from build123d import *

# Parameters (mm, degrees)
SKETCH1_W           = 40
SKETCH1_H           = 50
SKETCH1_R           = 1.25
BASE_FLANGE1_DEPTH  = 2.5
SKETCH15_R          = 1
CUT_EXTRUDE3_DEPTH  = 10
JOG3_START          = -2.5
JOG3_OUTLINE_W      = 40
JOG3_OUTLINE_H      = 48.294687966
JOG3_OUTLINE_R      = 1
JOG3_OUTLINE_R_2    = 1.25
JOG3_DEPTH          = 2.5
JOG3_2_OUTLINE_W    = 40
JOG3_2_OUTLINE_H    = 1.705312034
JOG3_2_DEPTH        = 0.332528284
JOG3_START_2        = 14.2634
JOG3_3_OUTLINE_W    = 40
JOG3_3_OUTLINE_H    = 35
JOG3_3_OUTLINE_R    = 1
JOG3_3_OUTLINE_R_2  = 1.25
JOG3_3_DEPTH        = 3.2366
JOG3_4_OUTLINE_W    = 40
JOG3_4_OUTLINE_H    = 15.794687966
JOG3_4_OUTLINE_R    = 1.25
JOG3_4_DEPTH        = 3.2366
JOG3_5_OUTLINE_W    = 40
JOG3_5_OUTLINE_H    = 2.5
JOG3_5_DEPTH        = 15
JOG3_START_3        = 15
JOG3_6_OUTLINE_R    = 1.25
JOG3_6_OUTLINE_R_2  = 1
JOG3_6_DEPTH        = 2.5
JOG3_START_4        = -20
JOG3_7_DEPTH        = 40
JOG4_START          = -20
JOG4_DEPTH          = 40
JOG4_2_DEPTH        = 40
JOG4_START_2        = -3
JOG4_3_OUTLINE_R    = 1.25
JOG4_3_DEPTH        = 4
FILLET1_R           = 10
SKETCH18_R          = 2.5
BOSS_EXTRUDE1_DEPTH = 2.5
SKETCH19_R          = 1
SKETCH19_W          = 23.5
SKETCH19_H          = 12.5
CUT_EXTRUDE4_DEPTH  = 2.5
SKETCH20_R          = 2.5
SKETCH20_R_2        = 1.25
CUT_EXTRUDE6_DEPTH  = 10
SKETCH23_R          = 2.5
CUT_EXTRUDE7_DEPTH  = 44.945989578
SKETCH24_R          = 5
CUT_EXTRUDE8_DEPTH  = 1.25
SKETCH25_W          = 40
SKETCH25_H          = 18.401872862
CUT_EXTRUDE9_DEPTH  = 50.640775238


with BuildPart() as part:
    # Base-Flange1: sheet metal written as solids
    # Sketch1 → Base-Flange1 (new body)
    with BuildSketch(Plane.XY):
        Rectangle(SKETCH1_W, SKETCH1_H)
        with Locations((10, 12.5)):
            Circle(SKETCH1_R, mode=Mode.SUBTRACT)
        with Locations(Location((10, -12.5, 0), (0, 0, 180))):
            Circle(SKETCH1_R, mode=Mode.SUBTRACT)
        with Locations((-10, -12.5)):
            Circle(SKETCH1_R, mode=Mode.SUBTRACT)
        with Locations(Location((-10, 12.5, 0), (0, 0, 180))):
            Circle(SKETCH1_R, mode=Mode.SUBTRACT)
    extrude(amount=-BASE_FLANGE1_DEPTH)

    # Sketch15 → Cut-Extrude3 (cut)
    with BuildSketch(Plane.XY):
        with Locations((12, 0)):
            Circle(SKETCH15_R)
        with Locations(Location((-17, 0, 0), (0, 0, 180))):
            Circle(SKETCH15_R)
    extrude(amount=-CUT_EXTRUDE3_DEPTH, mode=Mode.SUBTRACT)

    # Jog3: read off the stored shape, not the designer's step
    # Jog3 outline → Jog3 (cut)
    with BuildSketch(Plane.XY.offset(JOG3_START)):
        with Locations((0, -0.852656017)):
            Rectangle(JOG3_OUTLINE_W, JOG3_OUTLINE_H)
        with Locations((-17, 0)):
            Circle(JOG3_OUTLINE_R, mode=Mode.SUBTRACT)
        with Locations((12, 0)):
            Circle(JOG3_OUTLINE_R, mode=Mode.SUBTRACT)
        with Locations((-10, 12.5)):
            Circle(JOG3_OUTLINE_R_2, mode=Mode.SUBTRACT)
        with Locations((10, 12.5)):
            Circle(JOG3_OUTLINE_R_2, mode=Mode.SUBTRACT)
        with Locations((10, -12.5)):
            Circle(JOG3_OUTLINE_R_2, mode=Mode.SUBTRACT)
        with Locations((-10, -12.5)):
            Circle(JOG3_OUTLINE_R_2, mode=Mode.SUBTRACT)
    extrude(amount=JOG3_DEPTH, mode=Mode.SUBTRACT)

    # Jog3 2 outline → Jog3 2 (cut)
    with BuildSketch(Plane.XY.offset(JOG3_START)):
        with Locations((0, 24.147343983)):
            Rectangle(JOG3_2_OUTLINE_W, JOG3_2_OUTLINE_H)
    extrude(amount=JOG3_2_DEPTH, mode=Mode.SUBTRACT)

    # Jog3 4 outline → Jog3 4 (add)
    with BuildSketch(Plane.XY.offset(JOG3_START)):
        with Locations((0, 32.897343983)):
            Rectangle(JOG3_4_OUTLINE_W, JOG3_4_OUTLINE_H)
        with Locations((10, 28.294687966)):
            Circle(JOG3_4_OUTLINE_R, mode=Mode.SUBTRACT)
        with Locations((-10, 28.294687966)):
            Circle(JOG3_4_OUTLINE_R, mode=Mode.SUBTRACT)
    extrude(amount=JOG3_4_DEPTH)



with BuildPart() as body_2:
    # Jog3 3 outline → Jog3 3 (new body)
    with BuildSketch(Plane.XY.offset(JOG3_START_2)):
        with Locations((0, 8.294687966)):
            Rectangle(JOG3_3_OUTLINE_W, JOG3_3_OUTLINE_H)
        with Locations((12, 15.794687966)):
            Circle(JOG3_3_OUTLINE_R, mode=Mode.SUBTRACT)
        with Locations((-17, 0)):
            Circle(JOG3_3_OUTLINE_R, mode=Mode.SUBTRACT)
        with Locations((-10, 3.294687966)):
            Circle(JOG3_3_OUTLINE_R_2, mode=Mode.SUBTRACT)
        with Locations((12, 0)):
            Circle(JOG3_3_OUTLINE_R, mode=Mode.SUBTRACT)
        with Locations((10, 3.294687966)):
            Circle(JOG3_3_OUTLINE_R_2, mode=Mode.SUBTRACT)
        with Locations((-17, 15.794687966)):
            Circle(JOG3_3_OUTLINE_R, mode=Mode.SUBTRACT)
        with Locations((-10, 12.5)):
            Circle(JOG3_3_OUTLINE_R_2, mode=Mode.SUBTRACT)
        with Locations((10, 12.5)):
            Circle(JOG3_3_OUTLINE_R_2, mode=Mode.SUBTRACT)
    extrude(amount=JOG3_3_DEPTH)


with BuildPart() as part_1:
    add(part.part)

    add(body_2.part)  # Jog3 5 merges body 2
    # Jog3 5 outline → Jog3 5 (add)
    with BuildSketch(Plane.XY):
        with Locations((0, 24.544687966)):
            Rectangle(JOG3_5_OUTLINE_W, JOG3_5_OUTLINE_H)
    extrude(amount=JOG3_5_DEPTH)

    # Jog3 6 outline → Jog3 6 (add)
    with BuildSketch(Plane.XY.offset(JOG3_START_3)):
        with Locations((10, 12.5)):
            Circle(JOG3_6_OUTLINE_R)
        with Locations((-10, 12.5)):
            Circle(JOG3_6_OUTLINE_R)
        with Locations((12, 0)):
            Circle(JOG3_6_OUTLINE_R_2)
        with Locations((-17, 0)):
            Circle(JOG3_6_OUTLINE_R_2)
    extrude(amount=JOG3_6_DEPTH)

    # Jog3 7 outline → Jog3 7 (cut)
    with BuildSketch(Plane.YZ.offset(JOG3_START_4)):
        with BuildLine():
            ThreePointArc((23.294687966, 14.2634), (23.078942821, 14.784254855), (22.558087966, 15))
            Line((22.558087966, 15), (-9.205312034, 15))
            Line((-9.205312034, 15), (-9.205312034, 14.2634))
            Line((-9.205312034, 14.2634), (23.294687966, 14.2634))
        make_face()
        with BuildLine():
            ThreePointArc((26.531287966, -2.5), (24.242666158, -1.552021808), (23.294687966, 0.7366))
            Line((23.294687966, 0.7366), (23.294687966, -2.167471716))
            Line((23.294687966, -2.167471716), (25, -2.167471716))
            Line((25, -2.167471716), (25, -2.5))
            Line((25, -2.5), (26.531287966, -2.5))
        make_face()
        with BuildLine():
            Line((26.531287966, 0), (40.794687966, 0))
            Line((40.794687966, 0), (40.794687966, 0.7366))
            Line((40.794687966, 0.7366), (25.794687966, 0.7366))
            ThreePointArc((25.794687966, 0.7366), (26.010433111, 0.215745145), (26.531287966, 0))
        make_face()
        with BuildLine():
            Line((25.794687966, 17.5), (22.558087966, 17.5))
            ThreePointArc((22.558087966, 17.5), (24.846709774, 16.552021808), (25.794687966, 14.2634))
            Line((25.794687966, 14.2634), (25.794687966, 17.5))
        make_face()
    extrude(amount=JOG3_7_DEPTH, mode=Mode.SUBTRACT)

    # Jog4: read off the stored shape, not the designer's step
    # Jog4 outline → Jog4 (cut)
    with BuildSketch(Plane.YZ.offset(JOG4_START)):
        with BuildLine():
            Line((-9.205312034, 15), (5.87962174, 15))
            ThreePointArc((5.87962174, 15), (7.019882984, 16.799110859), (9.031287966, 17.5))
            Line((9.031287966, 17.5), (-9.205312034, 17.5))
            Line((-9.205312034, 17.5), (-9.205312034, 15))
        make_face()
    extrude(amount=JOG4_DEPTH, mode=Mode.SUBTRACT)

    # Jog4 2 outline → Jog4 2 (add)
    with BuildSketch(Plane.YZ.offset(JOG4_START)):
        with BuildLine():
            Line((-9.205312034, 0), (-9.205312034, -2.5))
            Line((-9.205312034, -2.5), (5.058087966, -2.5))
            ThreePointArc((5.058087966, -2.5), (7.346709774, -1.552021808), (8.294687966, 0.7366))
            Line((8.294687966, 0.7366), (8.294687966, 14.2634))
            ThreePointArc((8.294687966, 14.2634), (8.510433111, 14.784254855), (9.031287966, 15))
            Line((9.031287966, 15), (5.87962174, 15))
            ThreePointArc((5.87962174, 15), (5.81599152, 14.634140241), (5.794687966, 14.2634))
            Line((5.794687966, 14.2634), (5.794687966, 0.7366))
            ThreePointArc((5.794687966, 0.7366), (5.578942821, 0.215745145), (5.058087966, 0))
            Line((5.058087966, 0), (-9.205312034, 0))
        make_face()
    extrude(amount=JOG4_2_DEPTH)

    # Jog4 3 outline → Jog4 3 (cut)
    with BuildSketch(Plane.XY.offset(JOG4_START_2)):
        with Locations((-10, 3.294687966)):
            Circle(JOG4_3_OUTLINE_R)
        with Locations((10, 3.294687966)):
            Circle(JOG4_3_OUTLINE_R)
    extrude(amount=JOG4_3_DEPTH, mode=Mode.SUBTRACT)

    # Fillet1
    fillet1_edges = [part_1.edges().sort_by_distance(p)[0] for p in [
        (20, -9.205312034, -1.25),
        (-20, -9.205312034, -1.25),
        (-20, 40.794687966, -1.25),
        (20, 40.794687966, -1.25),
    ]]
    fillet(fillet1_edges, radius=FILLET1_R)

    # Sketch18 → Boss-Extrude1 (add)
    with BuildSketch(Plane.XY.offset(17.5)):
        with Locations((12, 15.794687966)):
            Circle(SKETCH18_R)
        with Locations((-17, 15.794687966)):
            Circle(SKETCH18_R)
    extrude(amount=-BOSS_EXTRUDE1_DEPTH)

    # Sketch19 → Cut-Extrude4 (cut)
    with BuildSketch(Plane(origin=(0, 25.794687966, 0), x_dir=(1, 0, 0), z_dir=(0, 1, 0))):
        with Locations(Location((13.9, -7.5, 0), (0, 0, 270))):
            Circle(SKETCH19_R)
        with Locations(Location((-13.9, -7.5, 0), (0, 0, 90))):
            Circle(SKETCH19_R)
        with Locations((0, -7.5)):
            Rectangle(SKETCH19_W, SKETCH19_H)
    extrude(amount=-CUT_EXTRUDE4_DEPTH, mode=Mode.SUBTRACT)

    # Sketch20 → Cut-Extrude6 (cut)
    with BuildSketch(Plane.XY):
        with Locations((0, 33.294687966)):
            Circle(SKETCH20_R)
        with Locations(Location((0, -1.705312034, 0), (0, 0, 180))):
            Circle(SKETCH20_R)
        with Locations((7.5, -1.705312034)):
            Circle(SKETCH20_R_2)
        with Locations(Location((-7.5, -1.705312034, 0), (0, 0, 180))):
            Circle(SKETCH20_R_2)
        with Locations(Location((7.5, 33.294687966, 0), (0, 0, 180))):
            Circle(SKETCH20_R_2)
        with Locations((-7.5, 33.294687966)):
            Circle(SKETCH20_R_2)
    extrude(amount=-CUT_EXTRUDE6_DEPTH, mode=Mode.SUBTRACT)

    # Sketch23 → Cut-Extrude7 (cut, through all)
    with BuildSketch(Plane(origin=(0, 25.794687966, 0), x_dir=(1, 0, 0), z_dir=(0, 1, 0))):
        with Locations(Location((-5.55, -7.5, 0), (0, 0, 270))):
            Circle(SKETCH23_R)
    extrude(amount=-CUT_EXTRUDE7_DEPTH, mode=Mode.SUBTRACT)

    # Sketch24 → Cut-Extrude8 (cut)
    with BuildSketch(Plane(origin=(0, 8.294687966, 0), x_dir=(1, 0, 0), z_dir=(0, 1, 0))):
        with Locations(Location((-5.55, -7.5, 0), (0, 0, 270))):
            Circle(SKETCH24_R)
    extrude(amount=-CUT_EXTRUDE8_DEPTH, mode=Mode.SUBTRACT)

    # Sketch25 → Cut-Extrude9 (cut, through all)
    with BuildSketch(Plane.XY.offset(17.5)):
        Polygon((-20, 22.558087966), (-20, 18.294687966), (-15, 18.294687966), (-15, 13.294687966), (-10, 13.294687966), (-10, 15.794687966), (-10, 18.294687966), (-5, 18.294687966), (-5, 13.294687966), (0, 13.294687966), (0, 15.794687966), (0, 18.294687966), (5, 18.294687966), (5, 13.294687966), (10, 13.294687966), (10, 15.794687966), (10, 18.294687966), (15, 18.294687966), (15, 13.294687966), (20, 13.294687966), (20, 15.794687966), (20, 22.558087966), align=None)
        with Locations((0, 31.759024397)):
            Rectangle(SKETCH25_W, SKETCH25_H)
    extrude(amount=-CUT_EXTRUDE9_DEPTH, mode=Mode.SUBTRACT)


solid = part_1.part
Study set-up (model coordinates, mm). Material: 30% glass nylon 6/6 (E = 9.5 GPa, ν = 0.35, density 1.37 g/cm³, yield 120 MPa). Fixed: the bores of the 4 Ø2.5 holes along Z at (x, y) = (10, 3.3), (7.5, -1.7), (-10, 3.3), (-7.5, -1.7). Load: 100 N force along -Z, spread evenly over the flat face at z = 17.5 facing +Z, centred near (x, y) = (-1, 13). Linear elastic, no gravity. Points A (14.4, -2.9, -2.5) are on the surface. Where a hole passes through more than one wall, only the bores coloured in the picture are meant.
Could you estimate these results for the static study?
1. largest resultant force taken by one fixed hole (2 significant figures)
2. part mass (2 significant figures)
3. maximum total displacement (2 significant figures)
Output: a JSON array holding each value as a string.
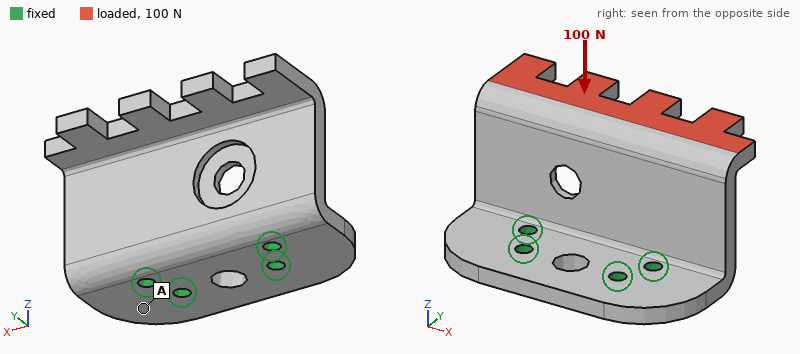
["81 N", "5.1 g", "0.53 mm"]
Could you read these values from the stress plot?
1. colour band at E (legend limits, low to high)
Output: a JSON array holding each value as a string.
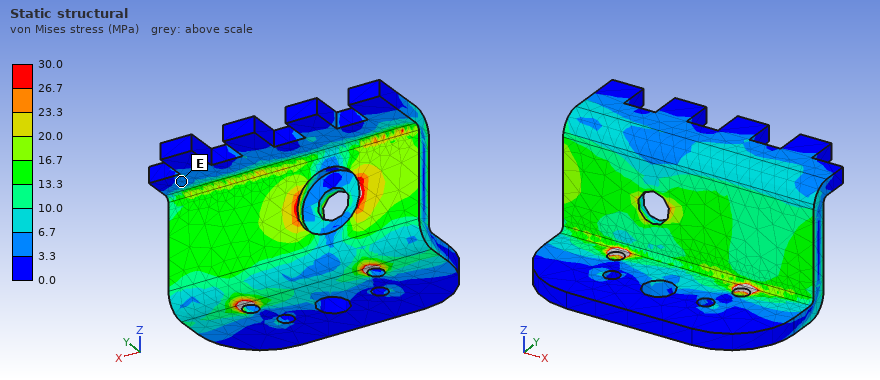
["3.3 to 6.7 MPa"]
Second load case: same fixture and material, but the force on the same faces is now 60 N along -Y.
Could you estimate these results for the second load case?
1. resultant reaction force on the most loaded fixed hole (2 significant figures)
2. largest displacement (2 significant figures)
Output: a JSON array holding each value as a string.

["45 N", "0.60 mm"]
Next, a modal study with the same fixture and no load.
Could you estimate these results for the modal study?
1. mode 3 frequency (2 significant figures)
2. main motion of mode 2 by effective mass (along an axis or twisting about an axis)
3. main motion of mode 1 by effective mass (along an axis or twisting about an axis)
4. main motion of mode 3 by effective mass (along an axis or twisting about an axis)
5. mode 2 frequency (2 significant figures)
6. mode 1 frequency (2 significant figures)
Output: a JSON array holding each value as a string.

["5800 Hz", "twisting about Z", "along Y", "along X", "2500 Hz", "1500 Hz"]
